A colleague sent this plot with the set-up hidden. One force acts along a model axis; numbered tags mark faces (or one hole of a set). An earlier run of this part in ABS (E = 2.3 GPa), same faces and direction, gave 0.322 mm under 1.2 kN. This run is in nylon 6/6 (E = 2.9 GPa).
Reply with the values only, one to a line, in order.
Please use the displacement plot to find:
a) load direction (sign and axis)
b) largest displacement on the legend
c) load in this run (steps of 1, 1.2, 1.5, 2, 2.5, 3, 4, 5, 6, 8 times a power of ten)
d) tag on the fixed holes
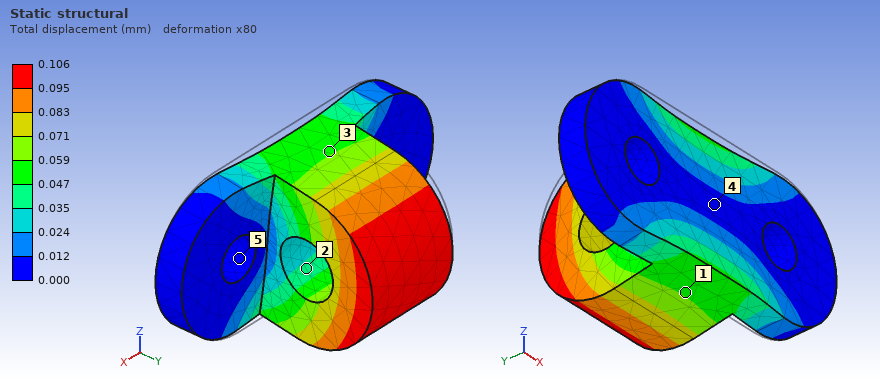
-Z
0.106 mm
500 N
5
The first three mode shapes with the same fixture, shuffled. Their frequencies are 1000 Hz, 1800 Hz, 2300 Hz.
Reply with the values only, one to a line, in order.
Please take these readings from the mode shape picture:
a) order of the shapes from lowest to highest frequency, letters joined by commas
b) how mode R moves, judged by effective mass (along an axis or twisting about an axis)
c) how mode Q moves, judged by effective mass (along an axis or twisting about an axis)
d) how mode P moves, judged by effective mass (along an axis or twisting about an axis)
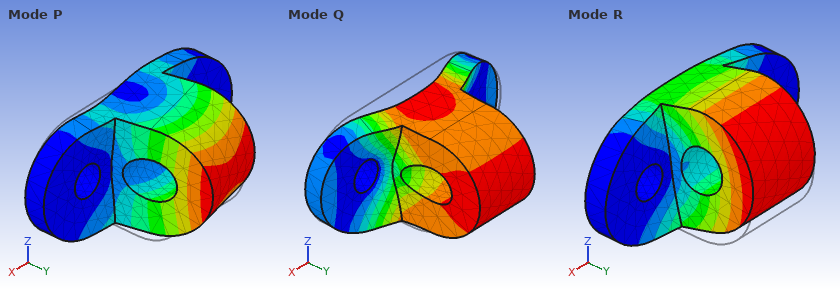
R, P, Q
along Z
along Y
along X
